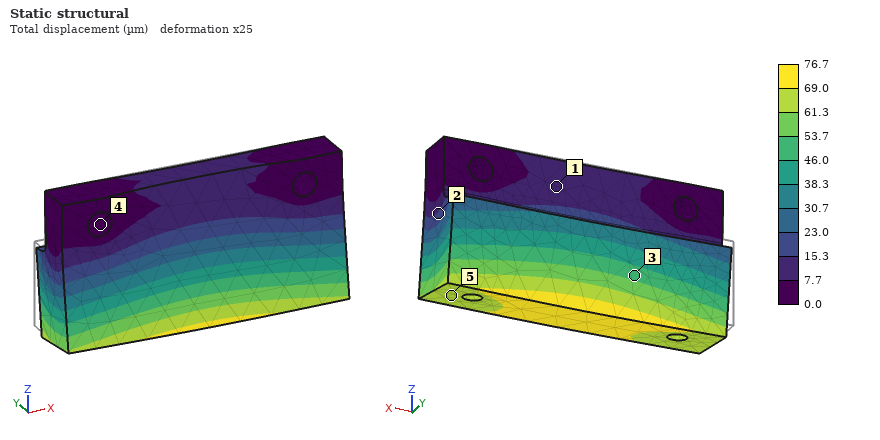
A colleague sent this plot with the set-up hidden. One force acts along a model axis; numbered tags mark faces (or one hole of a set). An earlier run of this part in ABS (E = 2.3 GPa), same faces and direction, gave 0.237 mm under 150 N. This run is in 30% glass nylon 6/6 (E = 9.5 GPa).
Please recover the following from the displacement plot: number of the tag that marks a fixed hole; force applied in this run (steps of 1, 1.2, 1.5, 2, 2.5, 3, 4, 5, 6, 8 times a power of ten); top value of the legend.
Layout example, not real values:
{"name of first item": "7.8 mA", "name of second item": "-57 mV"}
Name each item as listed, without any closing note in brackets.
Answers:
{"number of the tag that marks a fixed hole": "4", "force applied in this run": "200 N", "top value of the legend": "76.7 µm"}
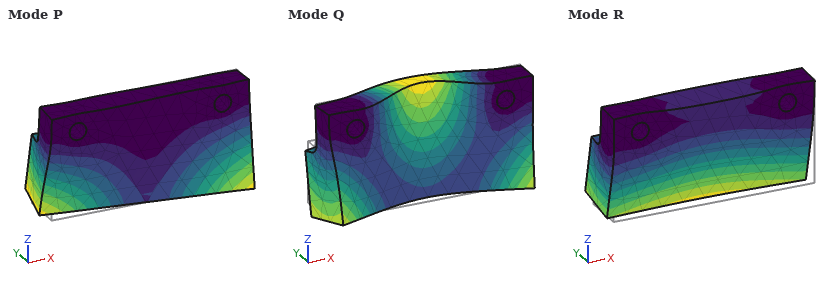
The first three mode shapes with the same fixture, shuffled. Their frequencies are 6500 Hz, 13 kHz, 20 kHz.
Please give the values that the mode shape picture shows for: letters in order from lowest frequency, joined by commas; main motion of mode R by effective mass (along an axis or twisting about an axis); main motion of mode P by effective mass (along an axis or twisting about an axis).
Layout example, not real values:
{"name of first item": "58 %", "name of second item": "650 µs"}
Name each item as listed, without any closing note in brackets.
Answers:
{"letters in order from lowest frequency, joined by commas": "R, P, Q", "main motion of mode R by effective mass": "along Y", "main motion of mode P by effective mass": "twisting about Z"}
